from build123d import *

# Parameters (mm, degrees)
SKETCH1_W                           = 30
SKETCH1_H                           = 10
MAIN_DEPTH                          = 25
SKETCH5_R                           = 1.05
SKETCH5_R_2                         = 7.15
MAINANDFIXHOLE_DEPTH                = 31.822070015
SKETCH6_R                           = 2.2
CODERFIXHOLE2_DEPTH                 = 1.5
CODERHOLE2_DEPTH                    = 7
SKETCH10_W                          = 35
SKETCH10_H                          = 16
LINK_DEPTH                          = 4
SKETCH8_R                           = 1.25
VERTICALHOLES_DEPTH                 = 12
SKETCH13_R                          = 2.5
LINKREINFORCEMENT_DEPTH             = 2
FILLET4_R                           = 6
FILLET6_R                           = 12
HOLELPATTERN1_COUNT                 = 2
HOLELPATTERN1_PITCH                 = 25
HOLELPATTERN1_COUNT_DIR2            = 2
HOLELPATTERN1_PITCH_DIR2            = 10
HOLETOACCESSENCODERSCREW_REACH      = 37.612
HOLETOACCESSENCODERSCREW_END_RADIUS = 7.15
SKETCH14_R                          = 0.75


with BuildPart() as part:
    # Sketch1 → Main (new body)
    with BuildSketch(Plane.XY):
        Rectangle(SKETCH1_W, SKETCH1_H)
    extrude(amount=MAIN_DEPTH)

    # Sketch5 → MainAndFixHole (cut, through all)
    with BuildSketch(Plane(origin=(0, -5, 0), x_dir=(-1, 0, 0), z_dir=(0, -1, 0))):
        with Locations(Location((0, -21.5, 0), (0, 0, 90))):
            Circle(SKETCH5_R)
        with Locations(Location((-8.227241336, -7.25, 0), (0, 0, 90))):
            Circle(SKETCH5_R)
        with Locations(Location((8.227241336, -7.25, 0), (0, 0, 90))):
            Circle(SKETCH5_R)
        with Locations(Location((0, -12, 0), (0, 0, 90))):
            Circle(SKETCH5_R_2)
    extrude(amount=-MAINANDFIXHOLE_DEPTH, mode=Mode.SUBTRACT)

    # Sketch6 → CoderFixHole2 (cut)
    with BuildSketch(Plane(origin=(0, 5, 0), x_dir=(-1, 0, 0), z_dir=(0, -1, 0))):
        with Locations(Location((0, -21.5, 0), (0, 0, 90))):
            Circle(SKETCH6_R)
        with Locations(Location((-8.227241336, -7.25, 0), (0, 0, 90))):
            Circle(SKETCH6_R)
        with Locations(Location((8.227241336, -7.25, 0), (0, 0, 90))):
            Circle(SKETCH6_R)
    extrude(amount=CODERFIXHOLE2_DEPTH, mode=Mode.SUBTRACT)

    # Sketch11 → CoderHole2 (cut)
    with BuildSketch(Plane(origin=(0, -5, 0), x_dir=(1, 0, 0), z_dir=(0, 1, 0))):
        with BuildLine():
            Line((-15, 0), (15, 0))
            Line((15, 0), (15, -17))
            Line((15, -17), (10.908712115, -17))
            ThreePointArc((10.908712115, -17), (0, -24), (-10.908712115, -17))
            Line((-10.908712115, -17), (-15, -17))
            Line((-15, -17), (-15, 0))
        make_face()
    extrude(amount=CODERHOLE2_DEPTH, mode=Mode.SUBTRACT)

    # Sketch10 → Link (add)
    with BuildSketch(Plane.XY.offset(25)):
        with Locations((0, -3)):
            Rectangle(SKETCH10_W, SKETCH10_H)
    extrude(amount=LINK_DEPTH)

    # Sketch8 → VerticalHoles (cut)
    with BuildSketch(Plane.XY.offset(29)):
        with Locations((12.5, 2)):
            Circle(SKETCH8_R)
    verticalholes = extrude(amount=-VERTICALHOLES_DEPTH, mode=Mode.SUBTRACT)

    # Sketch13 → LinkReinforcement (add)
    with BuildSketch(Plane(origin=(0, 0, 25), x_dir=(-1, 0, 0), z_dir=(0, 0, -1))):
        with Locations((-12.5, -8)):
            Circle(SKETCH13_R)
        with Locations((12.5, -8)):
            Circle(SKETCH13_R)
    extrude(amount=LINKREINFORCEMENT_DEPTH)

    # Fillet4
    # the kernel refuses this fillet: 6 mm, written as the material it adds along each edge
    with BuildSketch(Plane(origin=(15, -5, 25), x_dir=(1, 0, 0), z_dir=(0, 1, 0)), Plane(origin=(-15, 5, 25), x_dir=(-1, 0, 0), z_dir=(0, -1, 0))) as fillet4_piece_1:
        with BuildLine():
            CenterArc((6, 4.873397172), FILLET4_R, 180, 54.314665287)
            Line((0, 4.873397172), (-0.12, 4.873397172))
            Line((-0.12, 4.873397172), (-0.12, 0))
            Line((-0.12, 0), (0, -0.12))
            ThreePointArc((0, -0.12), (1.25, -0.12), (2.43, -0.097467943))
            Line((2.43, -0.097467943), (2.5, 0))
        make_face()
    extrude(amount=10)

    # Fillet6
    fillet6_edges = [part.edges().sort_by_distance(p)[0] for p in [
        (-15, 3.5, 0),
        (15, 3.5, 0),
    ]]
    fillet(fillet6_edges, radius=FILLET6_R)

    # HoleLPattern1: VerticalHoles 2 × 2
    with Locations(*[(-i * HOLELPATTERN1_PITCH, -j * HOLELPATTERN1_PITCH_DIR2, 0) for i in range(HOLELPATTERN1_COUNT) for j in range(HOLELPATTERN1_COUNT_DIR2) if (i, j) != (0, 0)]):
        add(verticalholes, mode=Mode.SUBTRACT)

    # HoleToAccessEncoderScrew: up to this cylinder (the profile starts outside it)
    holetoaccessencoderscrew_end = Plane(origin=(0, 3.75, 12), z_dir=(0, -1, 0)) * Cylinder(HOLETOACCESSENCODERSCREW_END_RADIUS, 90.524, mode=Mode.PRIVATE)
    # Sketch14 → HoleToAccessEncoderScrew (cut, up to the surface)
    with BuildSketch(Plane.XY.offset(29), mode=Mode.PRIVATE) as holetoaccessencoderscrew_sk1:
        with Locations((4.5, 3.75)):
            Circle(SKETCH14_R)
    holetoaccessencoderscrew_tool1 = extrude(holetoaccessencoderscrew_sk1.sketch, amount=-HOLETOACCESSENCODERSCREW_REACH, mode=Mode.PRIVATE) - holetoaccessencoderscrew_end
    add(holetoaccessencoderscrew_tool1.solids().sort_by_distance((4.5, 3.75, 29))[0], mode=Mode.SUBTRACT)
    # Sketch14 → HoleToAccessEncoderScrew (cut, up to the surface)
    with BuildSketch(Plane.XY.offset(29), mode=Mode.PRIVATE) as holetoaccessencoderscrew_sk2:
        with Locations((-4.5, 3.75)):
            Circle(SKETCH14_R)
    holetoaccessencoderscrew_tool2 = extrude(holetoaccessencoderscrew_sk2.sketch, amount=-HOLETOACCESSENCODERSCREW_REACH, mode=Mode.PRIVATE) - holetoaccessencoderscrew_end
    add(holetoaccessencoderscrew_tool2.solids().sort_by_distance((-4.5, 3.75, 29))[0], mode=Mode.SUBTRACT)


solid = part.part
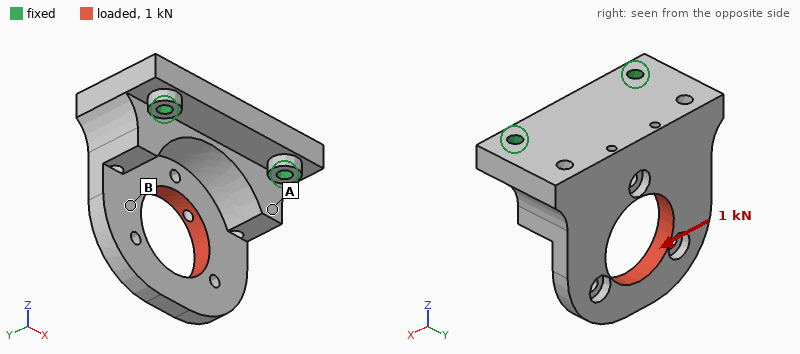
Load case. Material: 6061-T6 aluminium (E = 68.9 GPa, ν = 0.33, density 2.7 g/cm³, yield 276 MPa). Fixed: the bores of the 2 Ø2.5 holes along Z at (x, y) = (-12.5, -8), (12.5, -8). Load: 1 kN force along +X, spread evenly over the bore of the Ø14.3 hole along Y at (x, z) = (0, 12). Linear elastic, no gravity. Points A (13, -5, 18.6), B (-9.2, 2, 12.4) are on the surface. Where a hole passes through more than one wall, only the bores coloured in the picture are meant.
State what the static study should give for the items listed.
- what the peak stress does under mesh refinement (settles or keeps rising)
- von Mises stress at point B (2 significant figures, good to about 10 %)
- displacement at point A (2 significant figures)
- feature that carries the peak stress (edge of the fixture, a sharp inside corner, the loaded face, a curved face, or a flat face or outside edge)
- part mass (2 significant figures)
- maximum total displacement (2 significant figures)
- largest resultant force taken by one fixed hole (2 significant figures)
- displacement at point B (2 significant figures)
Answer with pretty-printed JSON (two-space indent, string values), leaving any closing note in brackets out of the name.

{
  "what the peak stress does under mesh refinement": "keeps rising",
  "von Mises stress at point B": "45 MPa",
  "displacement at point A": "15 µm",
  "feature that carries the peak stress": "edge of the fixture",
  "part mass": "12 g",
  "maximum total displacement": "65 µm",
  "largest resultant force taken by one fixed hole": "830 N",
  "displacement at point B": "38 µm"
}
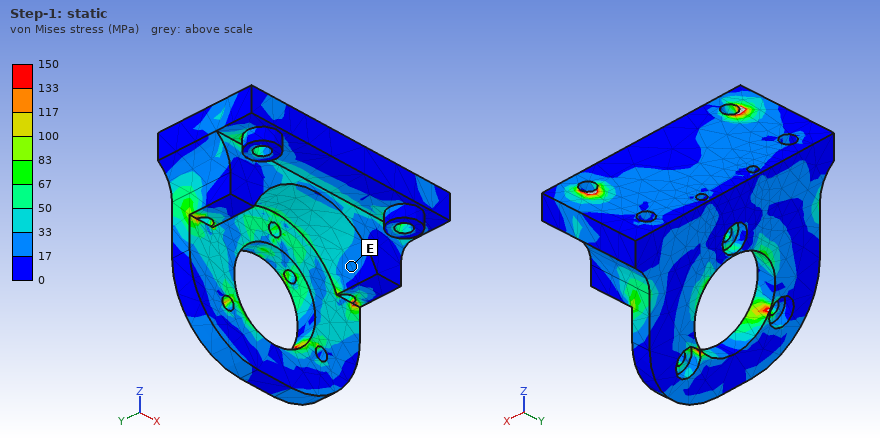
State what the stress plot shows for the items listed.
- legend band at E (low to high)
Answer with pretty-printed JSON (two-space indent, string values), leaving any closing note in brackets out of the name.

{
  "legend band at E": "17 to 33 MPa"
}
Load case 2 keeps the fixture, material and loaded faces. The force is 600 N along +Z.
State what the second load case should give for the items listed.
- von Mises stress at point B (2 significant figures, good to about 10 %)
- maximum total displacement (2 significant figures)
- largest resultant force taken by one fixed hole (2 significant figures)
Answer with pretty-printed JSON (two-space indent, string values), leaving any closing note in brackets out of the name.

{
  "von Mises stress at point B": "14 MPa",
  "maximum total displacement": "94 µm",
  "largest resultant force taken by one fixed hole": "300 N"
}
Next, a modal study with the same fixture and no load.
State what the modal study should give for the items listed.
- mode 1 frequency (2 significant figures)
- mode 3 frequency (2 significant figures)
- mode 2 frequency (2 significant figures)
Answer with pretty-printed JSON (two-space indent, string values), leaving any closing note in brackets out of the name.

{
  "mode 1 frequency": "4300 Hz",
  "mode 3 frequency": "10 kHz",
  "mode 2 frequency": "9600 Hz"
}
